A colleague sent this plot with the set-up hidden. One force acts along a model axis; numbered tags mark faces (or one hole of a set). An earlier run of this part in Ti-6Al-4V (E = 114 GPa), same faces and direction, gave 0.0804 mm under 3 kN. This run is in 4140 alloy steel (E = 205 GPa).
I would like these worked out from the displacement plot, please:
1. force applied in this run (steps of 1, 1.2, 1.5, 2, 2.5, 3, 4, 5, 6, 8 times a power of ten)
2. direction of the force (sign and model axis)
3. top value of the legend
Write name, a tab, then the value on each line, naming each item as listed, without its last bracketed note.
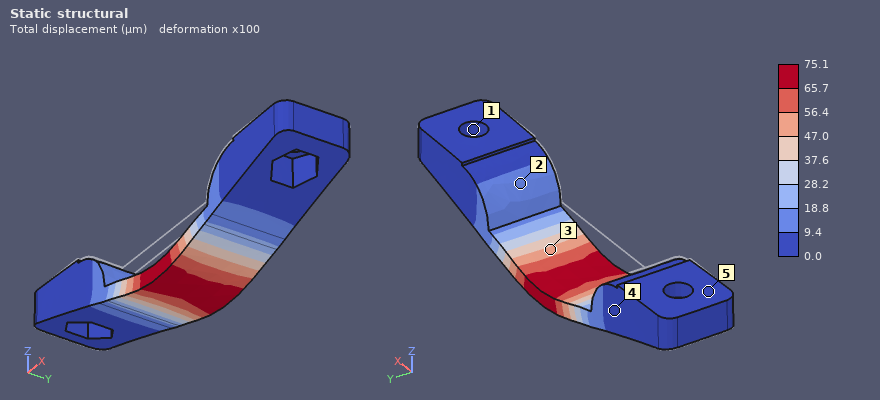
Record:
force applied in this run	5 kN
direction of the force	-Z
top value of the legend	75.1 µm
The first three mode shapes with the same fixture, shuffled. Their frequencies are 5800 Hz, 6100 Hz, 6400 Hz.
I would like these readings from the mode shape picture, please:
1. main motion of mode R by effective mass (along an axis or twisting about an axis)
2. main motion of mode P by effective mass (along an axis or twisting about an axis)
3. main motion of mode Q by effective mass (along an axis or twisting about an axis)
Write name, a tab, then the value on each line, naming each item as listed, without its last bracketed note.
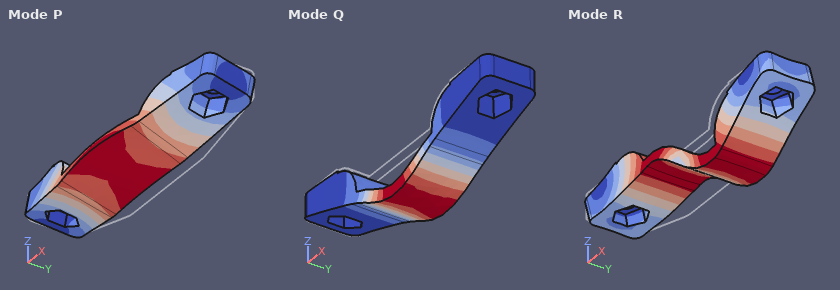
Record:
main motion of mode R by effective mass	along X
main motion of mode P by effective mass	along Y
main motion of mode Q by effective mass	along Z
